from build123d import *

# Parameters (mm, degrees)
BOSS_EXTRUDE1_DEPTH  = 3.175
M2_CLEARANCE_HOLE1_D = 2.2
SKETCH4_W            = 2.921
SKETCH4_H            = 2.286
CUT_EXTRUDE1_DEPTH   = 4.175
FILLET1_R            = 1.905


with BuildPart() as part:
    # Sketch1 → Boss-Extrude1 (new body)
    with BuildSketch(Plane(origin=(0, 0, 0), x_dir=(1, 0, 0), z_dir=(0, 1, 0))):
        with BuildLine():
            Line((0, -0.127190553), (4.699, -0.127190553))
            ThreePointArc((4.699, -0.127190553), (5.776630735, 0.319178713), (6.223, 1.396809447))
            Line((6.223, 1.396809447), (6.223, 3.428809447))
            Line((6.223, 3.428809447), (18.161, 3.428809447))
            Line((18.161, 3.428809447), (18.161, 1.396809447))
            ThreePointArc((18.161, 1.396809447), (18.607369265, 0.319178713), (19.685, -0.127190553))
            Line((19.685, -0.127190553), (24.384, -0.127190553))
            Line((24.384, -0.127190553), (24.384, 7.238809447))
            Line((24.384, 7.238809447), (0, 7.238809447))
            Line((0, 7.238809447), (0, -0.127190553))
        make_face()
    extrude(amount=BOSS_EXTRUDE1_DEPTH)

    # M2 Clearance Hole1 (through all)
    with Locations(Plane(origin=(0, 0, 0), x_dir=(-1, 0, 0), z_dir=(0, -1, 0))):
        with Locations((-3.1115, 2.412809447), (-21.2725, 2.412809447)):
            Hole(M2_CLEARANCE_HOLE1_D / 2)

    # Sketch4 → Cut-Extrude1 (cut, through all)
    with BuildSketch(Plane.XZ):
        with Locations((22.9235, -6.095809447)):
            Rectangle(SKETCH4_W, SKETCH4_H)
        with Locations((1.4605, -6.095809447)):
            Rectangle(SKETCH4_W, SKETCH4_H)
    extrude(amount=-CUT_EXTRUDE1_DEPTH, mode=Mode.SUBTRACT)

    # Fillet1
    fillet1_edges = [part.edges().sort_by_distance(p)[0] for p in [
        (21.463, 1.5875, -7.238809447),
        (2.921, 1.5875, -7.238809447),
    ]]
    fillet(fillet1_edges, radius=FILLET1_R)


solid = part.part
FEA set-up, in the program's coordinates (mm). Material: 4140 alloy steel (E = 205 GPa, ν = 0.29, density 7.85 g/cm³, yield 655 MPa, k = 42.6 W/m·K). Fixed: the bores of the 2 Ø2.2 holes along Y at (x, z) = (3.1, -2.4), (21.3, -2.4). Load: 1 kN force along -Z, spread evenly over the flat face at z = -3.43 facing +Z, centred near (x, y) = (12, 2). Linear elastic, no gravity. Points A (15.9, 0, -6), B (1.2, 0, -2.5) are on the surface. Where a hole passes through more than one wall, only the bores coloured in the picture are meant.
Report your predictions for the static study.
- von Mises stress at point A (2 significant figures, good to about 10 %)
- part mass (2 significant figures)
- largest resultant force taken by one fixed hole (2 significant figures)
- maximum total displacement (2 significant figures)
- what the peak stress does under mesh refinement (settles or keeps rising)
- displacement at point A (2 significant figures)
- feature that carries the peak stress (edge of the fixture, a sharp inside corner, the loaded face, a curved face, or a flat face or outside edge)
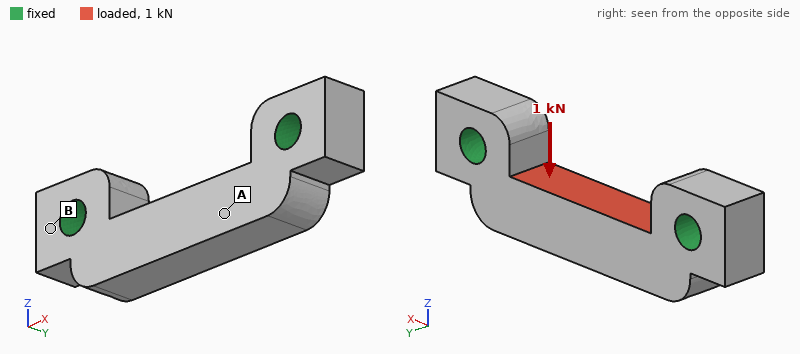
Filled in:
83 MPa
2.8 g
630 N
8.3 µm
keeps rising
5.6 µm
a sharp inside corner
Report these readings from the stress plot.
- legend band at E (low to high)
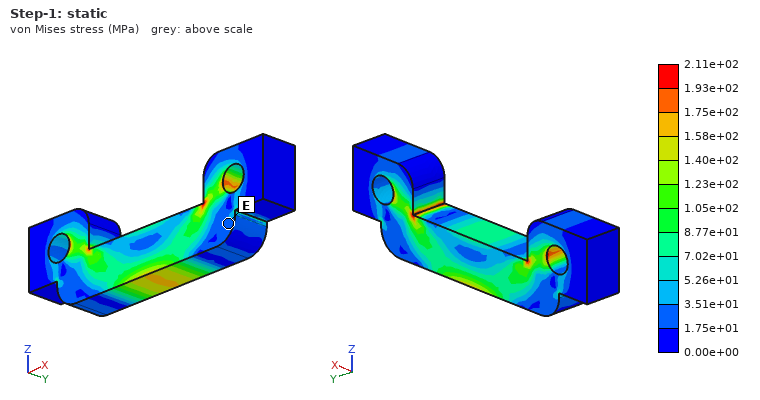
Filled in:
1.75e+01 to 3.51e+01 MPa
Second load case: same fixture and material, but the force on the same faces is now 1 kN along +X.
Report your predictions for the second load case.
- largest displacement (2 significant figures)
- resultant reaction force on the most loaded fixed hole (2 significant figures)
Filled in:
3.2 µm
500 N
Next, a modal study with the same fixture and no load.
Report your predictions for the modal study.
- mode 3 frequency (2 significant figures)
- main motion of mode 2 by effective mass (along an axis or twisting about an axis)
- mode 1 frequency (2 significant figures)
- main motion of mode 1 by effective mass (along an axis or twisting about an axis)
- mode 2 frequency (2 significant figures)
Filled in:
82 kHz
along Z
40 kHz
along Y
57 kHz
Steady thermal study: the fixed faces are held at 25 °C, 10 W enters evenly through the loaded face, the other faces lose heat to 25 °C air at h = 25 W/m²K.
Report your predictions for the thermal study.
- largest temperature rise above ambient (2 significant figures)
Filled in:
64 K
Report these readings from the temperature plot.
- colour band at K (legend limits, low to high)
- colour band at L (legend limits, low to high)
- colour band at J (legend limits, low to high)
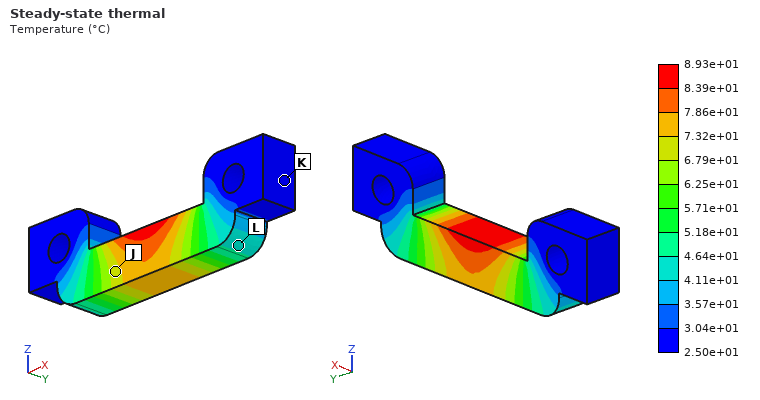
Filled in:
2.50e+01 to 3.04e+01 °C
4.11e+01 to 4.64e+01 °C
6.79e+01 to 7.32e+01 °C
